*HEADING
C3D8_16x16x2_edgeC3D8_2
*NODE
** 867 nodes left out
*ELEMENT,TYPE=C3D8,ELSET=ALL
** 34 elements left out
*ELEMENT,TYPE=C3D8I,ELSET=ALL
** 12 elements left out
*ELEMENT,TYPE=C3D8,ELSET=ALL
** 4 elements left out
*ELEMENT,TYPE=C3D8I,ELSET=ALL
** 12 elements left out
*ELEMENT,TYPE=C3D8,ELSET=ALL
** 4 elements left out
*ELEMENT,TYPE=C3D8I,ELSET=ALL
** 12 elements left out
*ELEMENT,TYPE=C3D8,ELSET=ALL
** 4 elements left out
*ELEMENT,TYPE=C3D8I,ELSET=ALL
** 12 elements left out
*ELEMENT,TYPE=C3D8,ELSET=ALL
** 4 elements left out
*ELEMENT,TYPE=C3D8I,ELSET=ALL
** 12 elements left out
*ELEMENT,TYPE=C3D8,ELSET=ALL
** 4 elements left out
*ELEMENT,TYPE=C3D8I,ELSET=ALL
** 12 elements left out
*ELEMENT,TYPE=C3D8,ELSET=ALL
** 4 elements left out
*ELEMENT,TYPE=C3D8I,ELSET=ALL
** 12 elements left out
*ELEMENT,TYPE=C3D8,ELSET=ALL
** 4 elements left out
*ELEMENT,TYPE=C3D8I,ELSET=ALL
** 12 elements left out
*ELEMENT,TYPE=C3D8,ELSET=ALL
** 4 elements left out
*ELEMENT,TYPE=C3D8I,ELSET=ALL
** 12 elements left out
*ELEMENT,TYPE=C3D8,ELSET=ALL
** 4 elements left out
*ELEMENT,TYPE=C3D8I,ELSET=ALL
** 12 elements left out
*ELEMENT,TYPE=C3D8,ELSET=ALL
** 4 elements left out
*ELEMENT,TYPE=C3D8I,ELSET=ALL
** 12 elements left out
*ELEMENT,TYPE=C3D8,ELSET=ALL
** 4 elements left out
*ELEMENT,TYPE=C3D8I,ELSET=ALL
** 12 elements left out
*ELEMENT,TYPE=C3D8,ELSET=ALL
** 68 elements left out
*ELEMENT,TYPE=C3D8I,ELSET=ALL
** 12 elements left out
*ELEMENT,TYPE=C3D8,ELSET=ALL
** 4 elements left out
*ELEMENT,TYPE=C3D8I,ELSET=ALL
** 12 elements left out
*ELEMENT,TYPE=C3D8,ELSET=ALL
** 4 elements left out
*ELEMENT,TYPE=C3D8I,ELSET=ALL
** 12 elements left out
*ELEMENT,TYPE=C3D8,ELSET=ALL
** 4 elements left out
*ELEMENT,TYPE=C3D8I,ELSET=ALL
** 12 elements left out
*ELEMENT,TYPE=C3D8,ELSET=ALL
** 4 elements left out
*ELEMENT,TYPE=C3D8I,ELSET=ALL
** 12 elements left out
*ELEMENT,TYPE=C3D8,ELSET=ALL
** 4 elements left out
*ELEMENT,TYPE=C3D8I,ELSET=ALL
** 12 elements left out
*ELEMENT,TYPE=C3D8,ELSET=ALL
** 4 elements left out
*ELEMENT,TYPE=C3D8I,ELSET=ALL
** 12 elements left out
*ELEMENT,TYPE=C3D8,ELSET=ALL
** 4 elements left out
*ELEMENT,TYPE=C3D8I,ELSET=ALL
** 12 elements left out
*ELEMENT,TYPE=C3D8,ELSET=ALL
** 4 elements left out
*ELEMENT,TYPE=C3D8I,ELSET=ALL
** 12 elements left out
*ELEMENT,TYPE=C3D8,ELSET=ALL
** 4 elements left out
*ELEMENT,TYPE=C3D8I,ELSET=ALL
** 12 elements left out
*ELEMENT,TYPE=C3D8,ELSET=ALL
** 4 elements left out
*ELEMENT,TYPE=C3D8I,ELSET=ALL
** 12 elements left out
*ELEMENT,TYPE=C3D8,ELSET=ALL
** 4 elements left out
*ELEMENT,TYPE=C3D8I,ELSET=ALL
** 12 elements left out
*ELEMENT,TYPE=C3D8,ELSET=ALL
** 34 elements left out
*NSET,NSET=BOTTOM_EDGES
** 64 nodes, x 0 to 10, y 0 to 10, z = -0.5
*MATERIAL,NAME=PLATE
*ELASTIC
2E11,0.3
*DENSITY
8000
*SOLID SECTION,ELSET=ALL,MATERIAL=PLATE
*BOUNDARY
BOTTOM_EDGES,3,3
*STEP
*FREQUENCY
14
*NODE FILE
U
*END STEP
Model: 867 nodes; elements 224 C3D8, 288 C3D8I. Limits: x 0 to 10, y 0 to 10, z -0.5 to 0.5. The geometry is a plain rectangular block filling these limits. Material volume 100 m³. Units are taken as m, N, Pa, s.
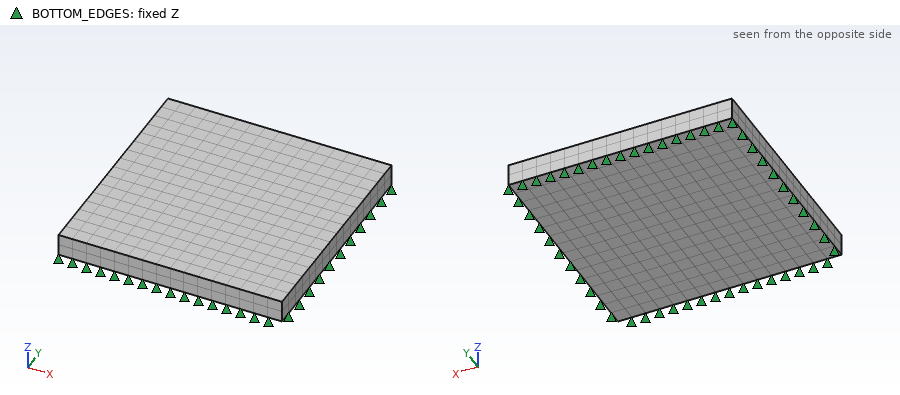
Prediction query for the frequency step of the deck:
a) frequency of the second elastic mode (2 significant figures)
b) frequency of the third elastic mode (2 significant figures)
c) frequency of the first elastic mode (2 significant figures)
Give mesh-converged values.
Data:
100 Hz
100 Hz
43 Hz
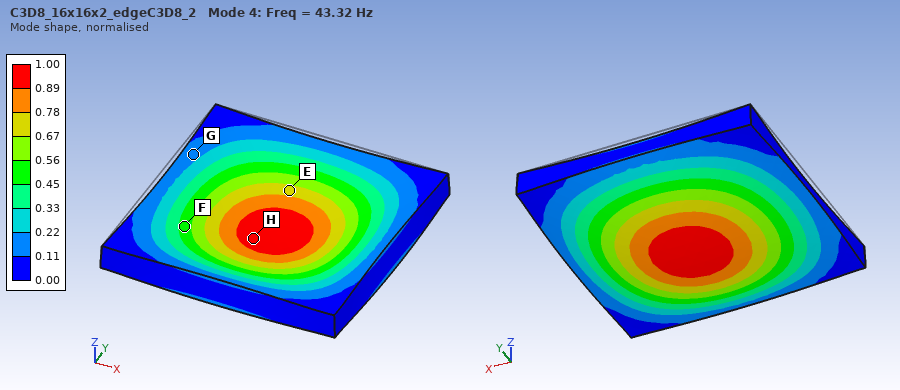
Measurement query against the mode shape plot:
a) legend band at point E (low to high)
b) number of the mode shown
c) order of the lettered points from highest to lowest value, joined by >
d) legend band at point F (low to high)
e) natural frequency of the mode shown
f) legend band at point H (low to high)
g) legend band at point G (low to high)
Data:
0.67 to 0.78
4
H > E > F > G
0.45 to 0.56
43.32 Hz
0.89 to 1.00
0.11 to 0.22
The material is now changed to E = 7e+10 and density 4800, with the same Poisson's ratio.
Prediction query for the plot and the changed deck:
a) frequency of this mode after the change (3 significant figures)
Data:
33.1 Hz
